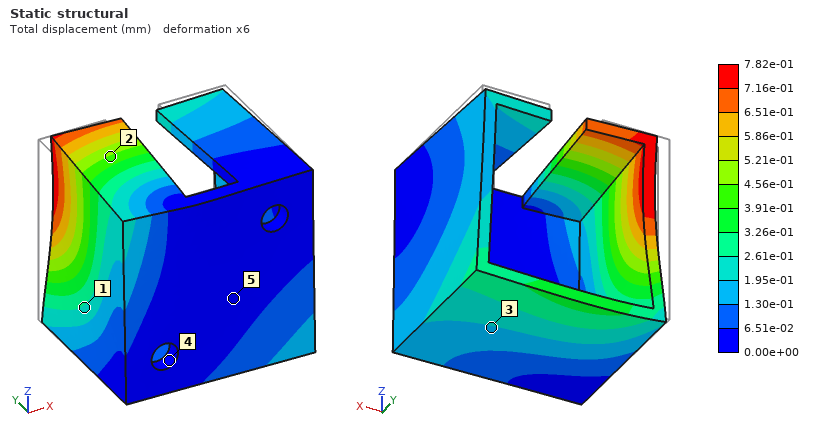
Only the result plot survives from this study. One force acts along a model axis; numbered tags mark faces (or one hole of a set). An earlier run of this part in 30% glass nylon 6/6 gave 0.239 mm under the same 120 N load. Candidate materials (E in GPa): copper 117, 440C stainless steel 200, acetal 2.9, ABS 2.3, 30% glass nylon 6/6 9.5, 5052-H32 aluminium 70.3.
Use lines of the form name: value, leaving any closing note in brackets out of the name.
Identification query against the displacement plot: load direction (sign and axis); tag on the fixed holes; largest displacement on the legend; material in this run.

load direction: +X
tag on the fixed holes: 4
largest displacement on the legend: 7.82e-01 mm
material in this run: acetal
